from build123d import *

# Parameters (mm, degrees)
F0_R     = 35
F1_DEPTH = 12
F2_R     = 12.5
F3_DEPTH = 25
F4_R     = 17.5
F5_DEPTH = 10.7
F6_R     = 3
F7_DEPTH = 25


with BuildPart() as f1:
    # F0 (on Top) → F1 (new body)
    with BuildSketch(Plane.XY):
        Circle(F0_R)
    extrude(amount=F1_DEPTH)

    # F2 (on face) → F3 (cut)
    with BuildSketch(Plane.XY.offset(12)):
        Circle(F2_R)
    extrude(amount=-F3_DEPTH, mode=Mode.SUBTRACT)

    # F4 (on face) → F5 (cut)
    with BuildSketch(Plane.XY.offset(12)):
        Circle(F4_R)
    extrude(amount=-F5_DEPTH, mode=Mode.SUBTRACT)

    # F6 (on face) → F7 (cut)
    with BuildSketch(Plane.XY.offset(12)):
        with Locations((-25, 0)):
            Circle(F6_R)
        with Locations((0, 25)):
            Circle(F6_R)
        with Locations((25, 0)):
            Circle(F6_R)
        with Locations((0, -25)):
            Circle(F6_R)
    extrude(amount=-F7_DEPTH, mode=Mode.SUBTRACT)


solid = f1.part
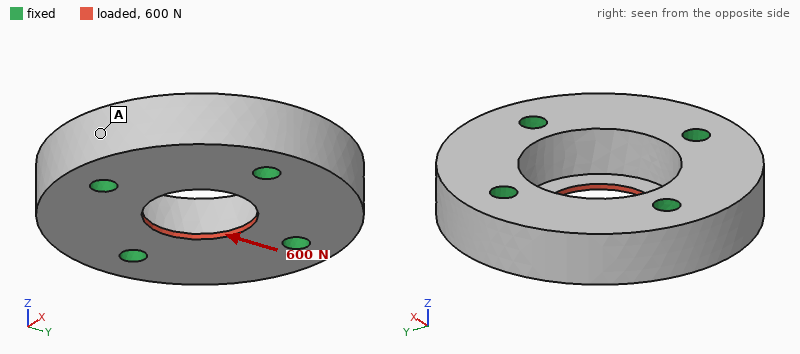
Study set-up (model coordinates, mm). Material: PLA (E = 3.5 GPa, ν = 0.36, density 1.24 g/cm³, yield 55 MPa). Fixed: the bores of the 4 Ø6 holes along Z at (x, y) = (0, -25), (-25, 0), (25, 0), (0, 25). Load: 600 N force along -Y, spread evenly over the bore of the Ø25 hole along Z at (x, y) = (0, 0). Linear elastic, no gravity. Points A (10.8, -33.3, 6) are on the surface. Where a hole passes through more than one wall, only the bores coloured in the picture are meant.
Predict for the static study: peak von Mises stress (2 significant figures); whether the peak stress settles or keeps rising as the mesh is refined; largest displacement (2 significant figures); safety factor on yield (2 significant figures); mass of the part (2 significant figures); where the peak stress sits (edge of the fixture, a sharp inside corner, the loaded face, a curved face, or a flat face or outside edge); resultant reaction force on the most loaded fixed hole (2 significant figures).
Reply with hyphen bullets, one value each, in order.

- 11 MPa
- settles
- 25 µm
- 5.0
- 42 g
- the loaded face
- 160 N
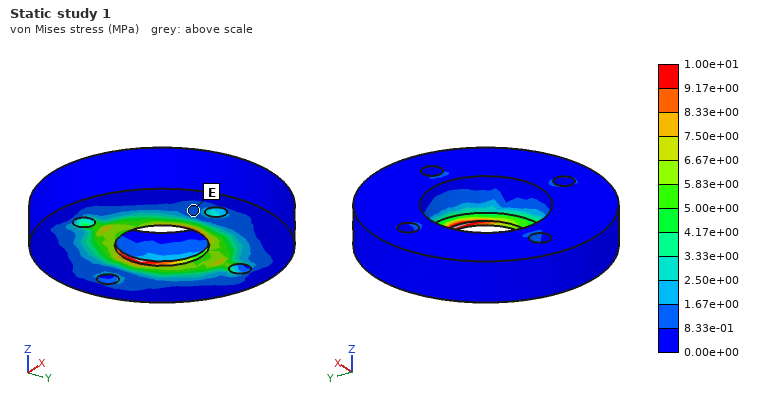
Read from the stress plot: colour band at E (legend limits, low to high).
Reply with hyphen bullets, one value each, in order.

- 8.33e-01 to 1.67e+00 MPa
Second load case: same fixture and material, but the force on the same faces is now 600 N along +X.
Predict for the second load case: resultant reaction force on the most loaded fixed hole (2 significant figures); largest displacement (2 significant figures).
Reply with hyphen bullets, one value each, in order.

- 160 N
- 25 µm
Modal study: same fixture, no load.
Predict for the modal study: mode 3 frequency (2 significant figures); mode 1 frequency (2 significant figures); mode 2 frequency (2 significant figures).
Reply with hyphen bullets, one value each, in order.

- 7500 Hz
- 7100 Hz
- 7500 Hz
